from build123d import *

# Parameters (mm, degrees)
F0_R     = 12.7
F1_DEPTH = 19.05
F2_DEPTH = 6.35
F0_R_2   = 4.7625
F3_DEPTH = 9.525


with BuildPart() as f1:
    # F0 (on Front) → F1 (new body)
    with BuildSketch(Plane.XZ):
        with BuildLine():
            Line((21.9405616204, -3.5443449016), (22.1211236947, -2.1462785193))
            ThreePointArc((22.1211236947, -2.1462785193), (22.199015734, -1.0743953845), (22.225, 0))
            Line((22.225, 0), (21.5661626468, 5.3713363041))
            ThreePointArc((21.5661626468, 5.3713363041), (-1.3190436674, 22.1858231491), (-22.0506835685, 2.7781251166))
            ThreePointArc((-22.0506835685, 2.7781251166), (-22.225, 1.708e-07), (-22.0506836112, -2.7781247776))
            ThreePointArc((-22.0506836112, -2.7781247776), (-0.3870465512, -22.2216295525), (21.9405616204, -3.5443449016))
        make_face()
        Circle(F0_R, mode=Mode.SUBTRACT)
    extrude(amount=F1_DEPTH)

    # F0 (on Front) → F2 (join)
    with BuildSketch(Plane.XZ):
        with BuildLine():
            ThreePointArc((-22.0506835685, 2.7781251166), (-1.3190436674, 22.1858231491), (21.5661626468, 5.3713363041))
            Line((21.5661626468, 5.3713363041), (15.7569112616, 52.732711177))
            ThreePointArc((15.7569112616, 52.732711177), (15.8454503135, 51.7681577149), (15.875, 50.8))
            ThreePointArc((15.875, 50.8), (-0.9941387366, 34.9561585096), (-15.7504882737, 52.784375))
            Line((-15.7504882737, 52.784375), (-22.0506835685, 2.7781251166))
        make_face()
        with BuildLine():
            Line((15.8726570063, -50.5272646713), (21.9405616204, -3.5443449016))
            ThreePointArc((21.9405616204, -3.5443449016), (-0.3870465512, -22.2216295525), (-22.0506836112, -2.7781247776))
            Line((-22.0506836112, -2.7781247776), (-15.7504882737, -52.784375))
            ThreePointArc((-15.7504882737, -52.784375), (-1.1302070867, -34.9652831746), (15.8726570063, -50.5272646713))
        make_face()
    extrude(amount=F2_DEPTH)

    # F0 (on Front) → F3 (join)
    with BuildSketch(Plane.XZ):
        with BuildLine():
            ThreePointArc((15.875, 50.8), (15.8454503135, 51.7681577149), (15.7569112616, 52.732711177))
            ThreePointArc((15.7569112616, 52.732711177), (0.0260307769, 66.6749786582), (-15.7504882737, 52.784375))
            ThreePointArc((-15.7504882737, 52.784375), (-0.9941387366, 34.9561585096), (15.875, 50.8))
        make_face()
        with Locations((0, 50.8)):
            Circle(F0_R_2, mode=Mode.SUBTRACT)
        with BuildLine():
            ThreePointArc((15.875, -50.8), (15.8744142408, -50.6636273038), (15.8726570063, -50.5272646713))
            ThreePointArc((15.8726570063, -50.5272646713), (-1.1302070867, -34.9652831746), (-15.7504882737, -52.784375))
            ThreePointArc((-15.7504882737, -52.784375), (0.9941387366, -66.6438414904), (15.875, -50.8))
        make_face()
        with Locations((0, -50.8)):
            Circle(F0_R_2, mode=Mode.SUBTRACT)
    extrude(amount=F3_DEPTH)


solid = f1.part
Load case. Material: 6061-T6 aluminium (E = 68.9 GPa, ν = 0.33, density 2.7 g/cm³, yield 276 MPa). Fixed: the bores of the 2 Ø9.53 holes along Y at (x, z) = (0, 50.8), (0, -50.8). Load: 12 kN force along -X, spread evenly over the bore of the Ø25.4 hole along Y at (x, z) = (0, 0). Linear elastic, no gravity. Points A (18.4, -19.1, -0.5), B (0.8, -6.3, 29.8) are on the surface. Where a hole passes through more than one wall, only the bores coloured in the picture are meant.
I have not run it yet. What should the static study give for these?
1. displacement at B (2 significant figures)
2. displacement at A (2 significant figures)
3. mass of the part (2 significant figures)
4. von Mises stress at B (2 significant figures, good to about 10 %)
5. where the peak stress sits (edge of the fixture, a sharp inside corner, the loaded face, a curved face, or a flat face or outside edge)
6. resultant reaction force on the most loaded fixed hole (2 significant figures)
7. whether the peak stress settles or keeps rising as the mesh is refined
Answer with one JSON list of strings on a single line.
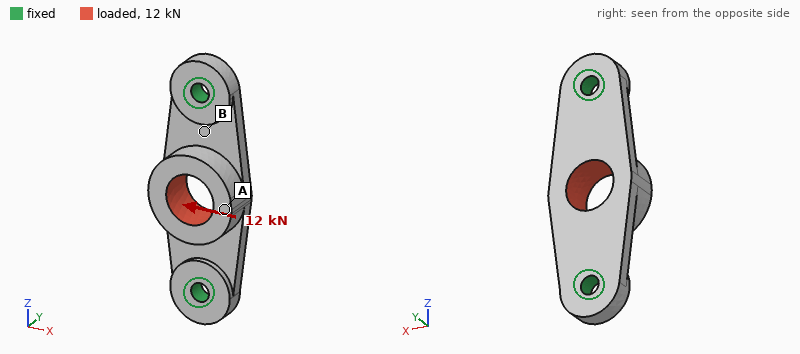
["0.053 mm", "0.26 mm", "120 g", "150 MPa", "edge of the fixture", "6.0 kN", "keeps rising"]
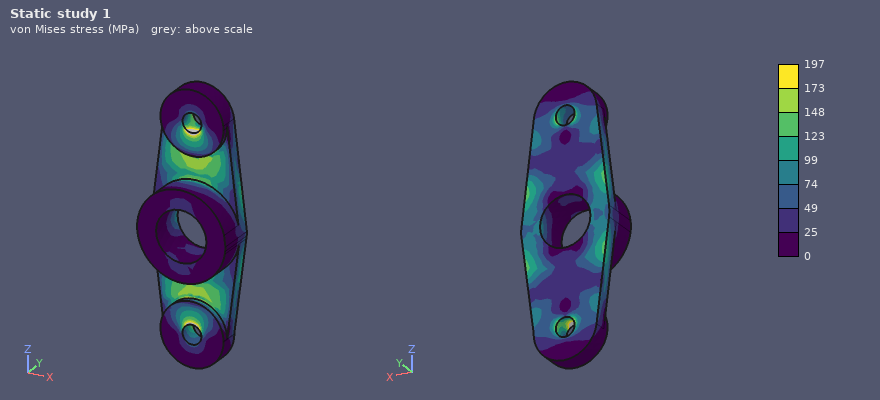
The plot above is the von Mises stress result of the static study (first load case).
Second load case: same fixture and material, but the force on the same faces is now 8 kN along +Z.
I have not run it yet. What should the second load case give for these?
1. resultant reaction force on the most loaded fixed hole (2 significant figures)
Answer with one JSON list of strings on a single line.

["4.1 kN"]
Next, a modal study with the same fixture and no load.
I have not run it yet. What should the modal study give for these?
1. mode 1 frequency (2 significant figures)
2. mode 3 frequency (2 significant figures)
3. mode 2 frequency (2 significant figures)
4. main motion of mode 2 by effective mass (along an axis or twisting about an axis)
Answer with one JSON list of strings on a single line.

["3800 Hz", "8500 Hz", "4200 Hz", "along Y"]
